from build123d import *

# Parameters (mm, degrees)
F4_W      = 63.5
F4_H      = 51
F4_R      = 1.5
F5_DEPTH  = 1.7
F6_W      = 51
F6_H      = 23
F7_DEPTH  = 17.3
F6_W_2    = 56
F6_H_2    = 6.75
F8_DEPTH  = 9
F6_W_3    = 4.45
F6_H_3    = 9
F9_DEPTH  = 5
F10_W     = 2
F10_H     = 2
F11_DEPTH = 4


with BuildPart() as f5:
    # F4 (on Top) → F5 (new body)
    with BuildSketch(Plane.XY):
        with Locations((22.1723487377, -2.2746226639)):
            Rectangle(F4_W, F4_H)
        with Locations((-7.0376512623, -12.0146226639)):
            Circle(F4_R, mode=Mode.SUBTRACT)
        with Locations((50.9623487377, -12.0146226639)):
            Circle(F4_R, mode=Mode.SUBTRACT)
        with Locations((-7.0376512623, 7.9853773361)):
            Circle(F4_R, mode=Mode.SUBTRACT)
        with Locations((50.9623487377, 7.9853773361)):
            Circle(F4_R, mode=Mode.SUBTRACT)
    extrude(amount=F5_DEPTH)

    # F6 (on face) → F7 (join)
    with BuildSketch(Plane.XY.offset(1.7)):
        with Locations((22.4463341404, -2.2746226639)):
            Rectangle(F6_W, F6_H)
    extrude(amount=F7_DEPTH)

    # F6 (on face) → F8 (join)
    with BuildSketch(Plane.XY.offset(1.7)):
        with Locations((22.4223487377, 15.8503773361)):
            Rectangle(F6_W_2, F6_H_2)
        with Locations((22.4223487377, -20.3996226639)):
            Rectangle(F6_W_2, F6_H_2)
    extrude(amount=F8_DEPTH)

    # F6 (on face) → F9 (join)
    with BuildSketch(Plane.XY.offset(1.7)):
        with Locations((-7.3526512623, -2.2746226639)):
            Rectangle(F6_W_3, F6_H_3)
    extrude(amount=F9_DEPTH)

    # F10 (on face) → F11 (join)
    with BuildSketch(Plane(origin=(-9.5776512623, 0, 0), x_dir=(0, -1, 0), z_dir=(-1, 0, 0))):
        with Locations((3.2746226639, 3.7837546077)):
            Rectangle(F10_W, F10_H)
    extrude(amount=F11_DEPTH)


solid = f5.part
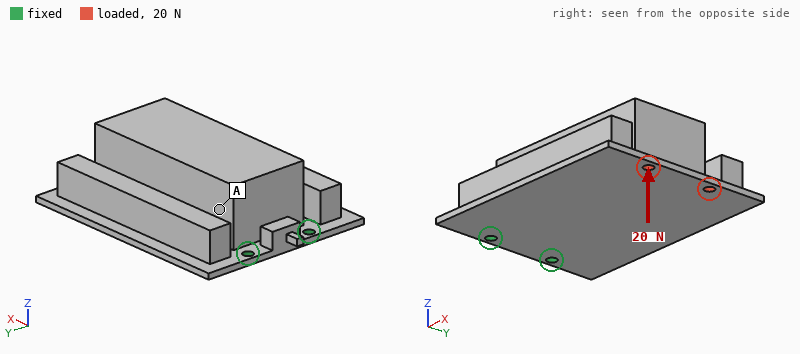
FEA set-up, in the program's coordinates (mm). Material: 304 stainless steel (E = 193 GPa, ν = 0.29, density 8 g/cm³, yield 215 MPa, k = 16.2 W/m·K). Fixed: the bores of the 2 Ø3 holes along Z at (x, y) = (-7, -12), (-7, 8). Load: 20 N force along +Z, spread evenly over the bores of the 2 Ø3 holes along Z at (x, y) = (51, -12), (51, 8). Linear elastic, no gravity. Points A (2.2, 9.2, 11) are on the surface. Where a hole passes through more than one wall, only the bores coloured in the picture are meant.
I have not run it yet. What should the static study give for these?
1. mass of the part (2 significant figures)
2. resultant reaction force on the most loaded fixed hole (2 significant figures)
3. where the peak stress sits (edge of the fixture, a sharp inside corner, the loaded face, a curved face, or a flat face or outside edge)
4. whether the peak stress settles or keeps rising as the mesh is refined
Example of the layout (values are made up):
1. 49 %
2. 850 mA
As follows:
1. 260 g
2. 11 N
3. edge of the fixture
4. keeps rising
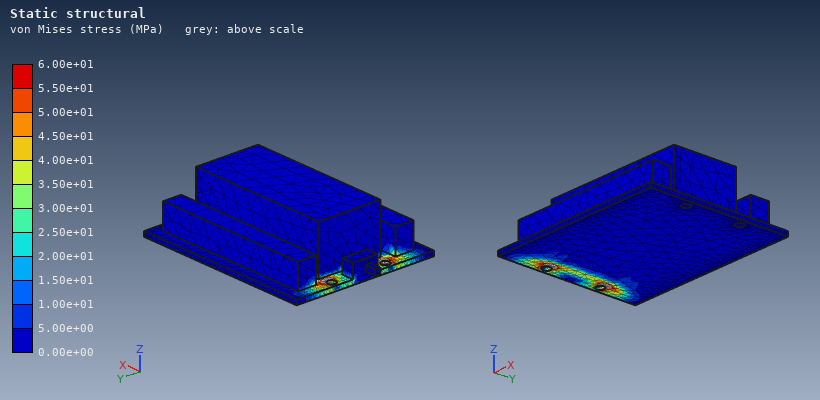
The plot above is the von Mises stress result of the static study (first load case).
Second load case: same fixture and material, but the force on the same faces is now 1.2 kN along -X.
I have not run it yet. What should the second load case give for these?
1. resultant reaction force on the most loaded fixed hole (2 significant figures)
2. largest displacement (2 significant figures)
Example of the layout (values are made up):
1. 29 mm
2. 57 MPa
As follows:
1. 600 N
2. 12 µm
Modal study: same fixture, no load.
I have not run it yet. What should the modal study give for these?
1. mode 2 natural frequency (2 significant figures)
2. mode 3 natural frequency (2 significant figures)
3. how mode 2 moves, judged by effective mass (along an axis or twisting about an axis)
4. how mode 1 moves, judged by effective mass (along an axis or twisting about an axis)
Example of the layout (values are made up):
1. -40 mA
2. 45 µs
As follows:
1. 2200 Hz
2. 2700 Hz
3. along Y
4. along Z
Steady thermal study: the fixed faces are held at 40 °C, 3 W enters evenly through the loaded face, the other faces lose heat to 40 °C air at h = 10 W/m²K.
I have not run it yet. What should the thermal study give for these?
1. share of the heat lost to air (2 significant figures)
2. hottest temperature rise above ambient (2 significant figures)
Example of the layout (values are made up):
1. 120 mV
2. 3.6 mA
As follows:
1. 57 %
2. 47 K
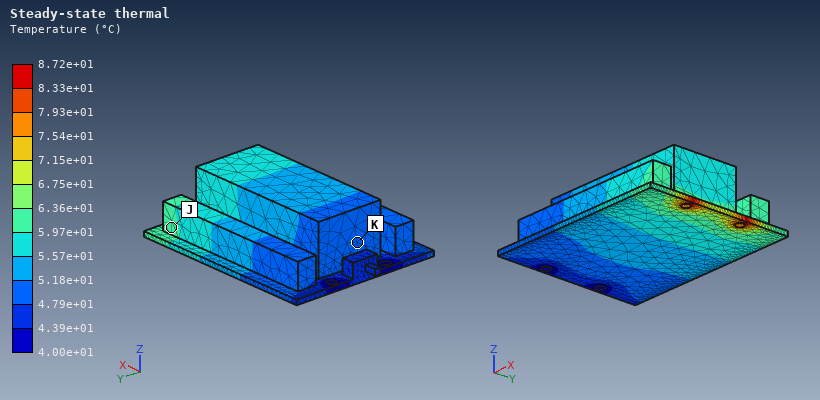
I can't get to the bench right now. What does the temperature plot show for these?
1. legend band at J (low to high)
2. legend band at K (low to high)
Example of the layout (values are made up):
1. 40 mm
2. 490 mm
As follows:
1. 5.97e+01 to 6.36e+01 °C
2. 4.79e+01 to 5.18e+01 °C
